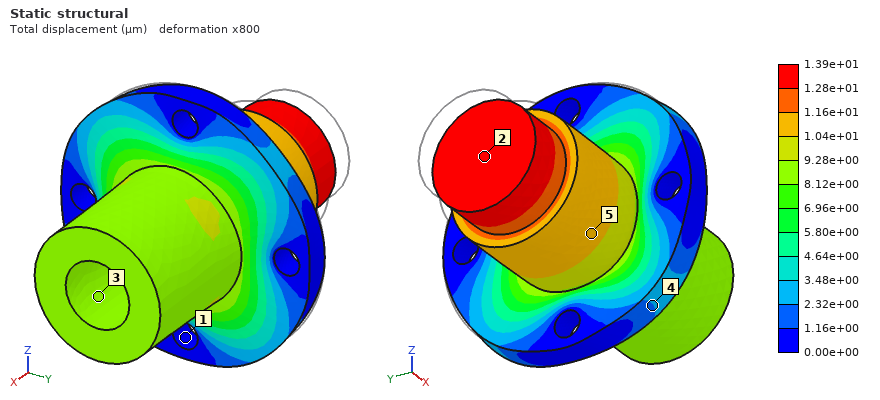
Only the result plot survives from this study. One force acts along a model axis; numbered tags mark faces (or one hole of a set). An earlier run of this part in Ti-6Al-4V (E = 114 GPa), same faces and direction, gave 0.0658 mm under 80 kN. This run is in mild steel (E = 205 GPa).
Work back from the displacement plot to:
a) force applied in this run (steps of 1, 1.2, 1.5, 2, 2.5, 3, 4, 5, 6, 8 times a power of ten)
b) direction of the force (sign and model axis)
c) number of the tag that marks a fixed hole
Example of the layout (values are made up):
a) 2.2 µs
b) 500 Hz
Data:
a) 30 kN
b) +X
c) 1
